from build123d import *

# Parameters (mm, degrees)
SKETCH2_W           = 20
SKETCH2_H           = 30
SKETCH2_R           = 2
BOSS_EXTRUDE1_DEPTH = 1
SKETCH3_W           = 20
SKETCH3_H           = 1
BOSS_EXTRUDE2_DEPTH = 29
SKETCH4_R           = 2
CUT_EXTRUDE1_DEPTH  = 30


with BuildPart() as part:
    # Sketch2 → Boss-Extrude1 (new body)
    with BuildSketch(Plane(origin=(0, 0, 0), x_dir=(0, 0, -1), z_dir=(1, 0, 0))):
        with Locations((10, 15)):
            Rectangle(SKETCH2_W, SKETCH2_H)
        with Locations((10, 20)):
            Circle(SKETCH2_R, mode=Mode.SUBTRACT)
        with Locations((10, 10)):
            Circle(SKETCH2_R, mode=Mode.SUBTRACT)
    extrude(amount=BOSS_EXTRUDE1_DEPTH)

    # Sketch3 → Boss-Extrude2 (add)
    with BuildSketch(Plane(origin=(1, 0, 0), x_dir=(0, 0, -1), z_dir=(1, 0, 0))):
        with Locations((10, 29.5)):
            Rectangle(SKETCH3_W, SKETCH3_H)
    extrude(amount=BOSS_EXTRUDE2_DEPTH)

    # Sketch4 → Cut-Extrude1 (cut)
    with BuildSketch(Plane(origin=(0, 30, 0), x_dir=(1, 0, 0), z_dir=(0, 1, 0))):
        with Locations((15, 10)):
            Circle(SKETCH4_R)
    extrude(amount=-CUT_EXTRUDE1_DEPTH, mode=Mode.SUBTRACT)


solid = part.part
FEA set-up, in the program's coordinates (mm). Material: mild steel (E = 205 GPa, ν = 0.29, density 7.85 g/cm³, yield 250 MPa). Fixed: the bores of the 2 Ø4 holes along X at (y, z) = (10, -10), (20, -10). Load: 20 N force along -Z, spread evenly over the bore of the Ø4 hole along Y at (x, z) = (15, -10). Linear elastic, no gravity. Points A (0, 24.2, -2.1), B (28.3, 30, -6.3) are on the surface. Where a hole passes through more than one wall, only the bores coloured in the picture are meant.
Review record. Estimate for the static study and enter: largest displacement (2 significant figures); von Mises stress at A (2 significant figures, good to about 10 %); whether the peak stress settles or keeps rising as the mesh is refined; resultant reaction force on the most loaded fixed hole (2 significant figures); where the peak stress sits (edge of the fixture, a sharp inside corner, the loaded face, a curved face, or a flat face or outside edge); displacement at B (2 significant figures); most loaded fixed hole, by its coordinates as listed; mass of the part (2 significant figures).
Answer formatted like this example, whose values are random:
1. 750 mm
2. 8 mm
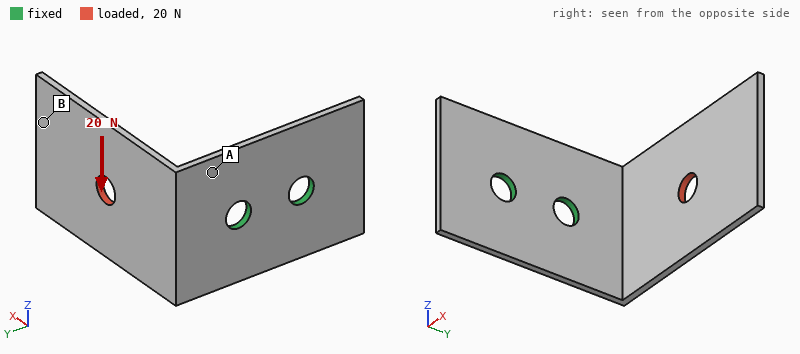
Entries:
1. 0.11 mm
2. 30 MPa
3. keeps rising
4. 31 N
5. edge of the fixture
6. 0.098 mm
7. (20, -10)
8. 9.0 g
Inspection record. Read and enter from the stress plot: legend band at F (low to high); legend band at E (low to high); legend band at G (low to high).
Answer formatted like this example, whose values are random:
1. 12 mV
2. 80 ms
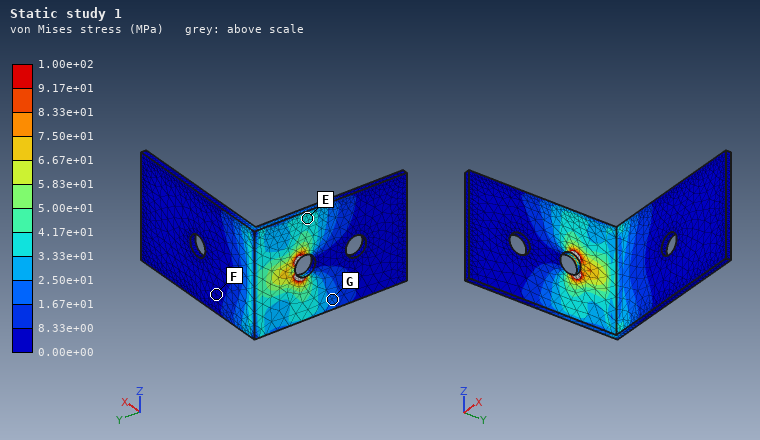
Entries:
1. 0.00e+00 to 8.33e+00 MPa
2. 3.33e+01 to 4.17e+01 MPa
3. 1.67e+01 to 2.50e+01 MPa
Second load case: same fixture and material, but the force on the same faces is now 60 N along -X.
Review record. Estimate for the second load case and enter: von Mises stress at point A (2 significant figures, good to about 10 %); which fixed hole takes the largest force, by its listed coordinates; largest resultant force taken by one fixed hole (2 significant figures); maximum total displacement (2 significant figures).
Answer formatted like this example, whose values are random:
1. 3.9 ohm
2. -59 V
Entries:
1. 66 MPa
2. (20, -10)
3. 70 N
4. 0.20 mm
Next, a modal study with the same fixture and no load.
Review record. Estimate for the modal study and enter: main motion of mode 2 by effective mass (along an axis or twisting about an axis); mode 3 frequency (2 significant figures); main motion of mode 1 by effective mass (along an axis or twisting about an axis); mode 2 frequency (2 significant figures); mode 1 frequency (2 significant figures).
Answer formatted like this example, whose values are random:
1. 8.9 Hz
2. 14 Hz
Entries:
1. along Z
2. 3000 Hz
3. along Y
4. 1200 Hz
5. 650 Hz
